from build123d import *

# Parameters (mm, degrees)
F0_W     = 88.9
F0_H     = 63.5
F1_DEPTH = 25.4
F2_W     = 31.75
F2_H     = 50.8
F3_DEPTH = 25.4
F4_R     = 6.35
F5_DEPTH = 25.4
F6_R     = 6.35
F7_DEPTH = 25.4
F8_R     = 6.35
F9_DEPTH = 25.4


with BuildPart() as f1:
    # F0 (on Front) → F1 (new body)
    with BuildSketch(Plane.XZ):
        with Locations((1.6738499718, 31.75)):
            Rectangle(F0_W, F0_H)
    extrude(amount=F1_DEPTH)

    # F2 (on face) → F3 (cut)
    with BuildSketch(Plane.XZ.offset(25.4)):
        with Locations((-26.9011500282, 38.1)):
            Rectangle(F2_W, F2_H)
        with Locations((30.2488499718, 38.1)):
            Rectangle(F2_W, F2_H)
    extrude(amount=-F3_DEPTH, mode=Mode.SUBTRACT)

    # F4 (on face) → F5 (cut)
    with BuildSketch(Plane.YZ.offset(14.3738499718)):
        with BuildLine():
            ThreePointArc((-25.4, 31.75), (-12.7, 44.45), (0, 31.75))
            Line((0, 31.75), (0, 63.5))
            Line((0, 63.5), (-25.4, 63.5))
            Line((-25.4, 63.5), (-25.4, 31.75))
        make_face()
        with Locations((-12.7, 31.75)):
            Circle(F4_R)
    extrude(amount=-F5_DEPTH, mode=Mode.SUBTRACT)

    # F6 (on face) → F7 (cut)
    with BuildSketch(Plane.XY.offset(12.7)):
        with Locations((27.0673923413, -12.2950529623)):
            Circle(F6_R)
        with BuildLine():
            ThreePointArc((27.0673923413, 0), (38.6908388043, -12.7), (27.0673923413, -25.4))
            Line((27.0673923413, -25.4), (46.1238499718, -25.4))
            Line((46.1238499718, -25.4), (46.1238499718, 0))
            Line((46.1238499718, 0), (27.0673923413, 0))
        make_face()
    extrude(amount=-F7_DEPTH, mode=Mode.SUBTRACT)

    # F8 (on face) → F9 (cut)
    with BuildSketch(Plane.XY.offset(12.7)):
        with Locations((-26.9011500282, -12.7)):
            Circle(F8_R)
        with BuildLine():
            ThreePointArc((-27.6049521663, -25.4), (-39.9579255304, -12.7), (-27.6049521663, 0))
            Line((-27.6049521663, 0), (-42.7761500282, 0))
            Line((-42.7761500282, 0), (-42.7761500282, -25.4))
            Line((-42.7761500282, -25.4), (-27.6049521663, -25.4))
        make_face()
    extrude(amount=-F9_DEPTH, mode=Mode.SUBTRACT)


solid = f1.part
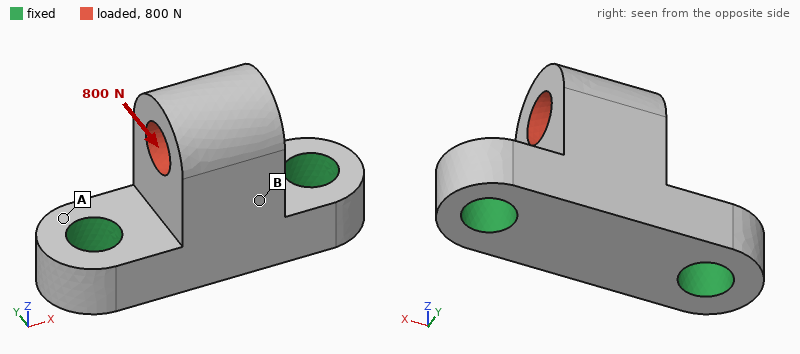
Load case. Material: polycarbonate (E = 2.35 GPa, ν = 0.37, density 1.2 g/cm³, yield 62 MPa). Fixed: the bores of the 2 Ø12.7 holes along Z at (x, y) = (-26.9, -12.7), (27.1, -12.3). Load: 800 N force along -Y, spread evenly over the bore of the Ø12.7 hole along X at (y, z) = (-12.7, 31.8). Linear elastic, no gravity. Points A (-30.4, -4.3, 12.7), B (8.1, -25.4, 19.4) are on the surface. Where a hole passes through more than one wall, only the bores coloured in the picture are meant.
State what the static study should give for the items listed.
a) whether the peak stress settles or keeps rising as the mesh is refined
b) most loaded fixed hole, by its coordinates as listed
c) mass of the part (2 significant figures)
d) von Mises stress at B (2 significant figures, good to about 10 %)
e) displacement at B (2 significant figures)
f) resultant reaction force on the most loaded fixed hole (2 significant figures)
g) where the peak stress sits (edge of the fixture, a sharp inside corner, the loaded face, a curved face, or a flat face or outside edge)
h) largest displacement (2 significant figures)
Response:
keeps rising
(27.1, -12.3)
43 g
4.7 MPa
0.25 mm
440 N
edge of the fixture
0.58 mm
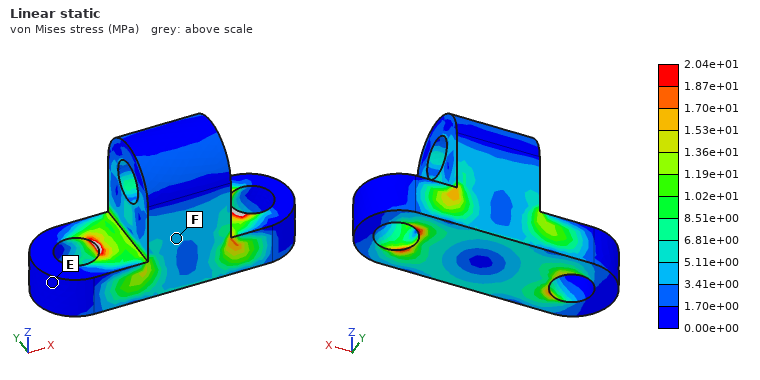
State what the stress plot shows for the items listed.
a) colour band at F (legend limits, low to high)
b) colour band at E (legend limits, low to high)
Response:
3.41e+00 to 5.11e+00 MPa
0.00e+00 to 1.70e+00 MPa
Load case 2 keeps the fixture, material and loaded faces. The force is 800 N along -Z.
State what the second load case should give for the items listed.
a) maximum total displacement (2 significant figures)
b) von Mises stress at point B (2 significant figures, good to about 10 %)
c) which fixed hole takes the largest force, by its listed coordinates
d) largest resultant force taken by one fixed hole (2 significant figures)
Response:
63 µm
1.5 MPa
(27.1, -12.3)
450 N
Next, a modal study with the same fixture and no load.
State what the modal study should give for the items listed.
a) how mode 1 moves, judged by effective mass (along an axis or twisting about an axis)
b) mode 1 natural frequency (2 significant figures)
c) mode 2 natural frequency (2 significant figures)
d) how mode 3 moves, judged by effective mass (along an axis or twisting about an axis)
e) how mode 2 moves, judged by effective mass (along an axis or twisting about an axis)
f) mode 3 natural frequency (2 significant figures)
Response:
along Y
1800 Hz
3200 Hz
along Z
along X
4300 Hz
